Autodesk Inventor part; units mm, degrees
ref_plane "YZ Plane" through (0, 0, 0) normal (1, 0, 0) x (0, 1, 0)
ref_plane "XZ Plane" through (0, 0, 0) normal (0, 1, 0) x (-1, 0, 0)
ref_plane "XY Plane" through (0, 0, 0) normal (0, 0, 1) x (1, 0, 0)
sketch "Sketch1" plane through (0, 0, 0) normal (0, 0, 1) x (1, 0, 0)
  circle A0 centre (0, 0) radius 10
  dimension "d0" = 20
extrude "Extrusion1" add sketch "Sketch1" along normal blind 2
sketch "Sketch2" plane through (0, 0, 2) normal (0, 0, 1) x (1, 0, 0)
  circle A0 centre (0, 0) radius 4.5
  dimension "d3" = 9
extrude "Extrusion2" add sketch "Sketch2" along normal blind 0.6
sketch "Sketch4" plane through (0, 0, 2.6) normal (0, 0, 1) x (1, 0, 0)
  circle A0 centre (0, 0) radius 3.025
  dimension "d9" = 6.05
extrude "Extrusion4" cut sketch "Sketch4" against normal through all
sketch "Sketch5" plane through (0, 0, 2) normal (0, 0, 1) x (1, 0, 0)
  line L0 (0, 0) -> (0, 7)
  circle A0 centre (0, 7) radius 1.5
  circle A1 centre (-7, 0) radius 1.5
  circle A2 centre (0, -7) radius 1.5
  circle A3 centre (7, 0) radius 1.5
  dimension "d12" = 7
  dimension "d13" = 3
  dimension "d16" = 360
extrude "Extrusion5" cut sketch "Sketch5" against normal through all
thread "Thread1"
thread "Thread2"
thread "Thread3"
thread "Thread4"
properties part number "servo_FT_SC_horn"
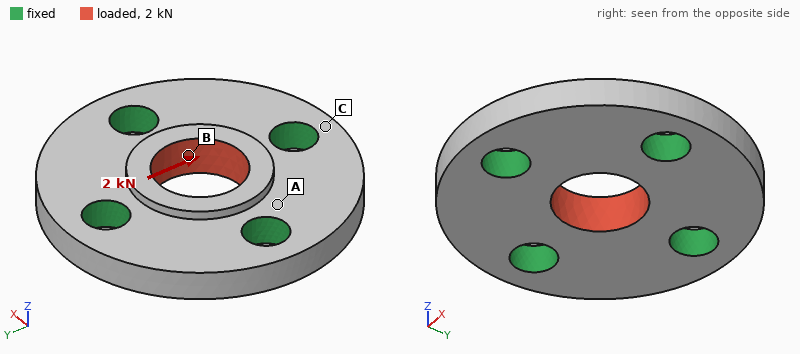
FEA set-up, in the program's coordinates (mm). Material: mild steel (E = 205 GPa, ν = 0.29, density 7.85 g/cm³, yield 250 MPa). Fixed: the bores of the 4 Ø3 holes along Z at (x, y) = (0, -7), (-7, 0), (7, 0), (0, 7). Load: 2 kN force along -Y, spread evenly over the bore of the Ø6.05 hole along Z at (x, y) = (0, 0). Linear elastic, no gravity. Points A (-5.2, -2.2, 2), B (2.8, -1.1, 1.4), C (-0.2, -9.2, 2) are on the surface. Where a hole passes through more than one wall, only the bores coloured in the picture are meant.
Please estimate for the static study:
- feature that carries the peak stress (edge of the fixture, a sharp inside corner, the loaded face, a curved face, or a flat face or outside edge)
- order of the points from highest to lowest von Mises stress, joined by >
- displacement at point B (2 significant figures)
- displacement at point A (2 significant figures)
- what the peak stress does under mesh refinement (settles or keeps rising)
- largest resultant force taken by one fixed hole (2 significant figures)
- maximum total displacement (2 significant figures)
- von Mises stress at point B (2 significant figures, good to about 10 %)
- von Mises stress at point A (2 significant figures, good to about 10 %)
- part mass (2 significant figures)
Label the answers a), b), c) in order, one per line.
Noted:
a) a sharp inside corner
b) B > A > C
c) 1.2 µm
d) 0.43 µm
e) keeps rising
f) 620 N
g) 1.4 µm
h) 70 MPa
i) 31 MPa
j) 4.2 g
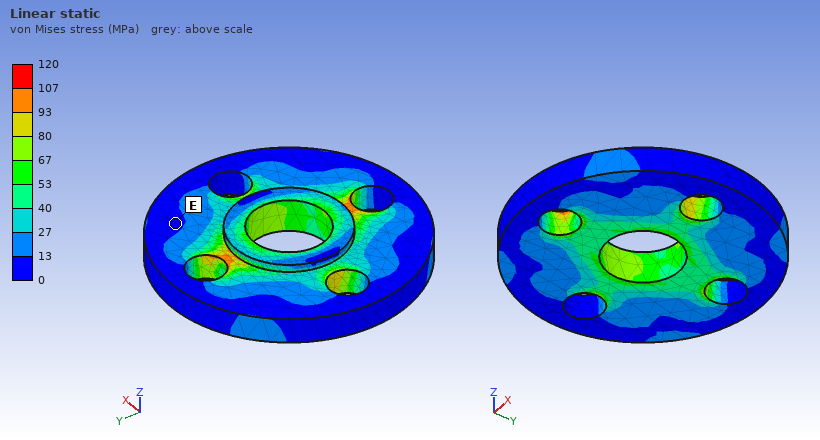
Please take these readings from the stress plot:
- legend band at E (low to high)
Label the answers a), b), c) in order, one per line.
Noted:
a) 0 to 13 MPa
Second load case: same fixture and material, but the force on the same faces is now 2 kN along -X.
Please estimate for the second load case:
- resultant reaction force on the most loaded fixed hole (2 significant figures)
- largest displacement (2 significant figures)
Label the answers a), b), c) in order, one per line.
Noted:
a) 620 N
b) 1.4 µm
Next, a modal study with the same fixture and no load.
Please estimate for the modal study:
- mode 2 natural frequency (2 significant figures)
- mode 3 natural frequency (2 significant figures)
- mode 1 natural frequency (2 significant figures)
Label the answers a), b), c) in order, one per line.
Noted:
a) 77 kHz
b) 77 kHz
c) 77 kHz
